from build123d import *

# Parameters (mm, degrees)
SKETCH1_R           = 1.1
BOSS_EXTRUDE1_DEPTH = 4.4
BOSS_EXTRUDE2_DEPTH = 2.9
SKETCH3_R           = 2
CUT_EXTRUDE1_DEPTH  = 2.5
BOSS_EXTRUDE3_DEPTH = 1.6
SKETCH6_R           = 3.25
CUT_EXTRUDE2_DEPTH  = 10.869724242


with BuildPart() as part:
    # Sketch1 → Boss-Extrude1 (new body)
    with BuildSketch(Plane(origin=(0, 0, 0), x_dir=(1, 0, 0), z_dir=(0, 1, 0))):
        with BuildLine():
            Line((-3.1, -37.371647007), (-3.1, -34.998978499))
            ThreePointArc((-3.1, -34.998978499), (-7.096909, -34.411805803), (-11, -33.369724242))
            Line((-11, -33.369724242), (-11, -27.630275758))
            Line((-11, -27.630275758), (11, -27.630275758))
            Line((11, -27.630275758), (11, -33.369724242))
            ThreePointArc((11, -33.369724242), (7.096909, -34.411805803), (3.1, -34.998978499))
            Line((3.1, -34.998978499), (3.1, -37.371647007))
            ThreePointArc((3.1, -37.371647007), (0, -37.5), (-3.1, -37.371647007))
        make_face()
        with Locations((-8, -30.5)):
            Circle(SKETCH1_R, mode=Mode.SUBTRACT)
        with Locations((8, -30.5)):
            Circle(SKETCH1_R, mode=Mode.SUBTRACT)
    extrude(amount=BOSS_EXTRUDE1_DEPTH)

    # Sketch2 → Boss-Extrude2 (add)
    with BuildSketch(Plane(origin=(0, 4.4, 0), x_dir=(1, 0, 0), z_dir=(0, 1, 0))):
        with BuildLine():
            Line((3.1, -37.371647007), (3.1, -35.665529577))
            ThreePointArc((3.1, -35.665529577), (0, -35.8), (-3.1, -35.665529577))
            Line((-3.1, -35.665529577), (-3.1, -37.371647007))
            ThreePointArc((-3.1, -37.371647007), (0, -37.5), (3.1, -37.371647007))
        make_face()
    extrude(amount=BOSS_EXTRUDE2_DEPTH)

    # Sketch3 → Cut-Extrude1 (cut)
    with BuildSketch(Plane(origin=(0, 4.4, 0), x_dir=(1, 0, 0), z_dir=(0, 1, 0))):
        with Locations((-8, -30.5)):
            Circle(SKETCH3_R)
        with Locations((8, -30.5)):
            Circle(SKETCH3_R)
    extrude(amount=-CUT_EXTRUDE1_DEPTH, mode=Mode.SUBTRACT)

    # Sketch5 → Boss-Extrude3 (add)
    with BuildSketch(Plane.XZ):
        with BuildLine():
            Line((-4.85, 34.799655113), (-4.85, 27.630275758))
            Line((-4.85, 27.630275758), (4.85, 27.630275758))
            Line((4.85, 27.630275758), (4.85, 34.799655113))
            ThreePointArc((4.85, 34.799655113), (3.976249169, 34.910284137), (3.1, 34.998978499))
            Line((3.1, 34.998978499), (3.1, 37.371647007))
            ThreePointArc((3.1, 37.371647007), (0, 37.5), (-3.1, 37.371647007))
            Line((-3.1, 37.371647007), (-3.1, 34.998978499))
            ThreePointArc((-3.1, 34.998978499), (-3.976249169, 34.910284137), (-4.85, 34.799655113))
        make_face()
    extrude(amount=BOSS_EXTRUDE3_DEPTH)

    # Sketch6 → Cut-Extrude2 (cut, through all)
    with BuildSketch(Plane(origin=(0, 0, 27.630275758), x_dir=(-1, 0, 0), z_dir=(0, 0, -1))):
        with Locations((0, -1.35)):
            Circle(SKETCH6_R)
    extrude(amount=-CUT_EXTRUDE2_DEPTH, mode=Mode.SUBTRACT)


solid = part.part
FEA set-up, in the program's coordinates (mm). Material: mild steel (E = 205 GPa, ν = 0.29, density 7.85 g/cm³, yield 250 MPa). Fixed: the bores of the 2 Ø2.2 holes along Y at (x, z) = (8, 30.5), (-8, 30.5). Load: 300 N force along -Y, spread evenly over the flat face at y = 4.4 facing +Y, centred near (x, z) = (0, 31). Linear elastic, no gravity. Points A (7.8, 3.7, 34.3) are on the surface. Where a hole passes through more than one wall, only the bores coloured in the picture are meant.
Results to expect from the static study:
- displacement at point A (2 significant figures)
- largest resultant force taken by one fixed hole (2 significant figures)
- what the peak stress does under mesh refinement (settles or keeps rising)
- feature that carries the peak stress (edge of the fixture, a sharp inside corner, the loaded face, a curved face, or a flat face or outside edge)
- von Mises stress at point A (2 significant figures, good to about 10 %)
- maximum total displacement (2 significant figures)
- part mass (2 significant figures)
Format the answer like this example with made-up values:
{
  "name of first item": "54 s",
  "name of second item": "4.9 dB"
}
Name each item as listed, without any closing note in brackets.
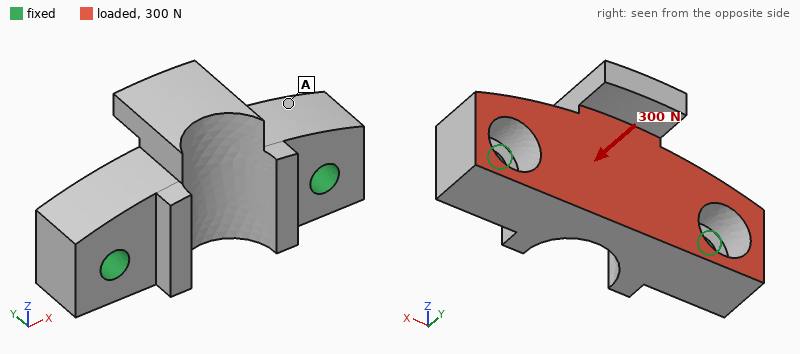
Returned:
{
  "displacement at point A": "0.66 µm",
  "largest resultant force taken by one fixed hole": "180 N",
  "what the peak stress does under mesh refinement": "keeps rising",
  "feature that carries the peak stress": "edge of the fixture",
  "von Mises stress at point A": "6.3 MPa",
  "maximum total displacement": "2.1 µm",
  "part mass": "5.1 g"
}
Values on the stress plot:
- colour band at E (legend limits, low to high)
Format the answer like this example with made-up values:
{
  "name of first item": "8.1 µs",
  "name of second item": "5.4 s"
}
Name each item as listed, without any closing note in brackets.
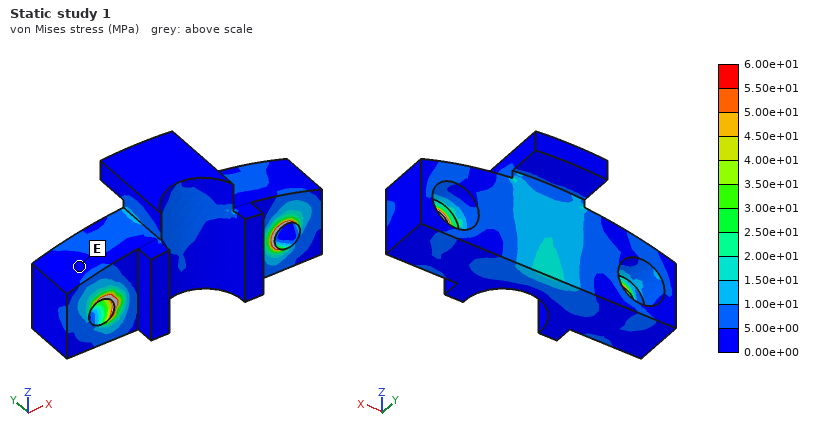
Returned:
{
  "colour band at E": "0.00e+00 to 5.00e+00 MPa"
}
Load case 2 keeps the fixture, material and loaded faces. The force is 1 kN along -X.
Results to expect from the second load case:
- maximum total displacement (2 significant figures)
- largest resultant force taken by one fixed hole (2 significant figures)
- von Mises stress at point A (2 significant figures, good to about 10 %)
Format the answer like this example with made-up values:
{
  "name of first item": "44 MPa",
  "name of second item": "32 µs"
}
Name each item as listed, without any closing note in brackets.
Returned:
{
  "maximum total displacement": "1.9 µm",
  "largest resultant force taken by one fixed hole": "540 N",
  "von Mises stress at point A": "11 MPa"
}
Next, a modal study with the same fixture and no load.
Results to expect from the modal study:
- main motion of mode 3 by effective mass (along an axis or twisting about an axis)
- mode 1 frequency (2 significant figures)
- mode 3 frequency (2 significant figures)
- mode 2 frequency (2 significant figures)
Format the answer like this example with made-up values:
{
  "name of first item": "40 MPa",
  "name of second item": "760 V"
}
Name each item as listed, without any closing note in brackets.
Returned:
{
  "main motion of mode 3 by effective mass": "along Z",
  "mode 1 frequency": "25 kHz",
  "mode 3 frequency": "61 kHz",
  "mode 2 frequency": "49 kHz"
}
